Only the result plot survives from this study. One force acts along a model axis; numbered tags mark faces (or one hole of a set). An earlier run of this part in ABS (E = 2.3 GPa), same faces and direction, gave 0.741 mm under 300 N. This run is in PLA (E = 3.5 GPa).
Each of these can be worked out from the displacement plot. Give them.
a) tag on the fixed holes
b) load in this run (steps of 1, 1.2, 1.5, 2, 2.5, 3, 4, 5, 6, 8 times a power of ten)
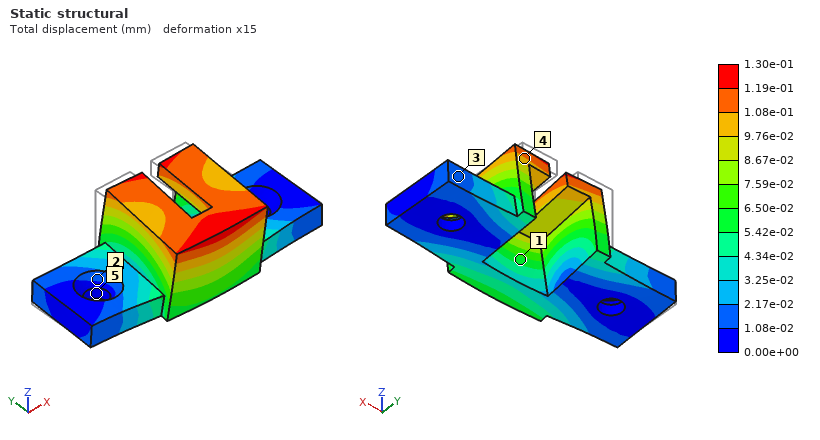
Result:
5
80 N
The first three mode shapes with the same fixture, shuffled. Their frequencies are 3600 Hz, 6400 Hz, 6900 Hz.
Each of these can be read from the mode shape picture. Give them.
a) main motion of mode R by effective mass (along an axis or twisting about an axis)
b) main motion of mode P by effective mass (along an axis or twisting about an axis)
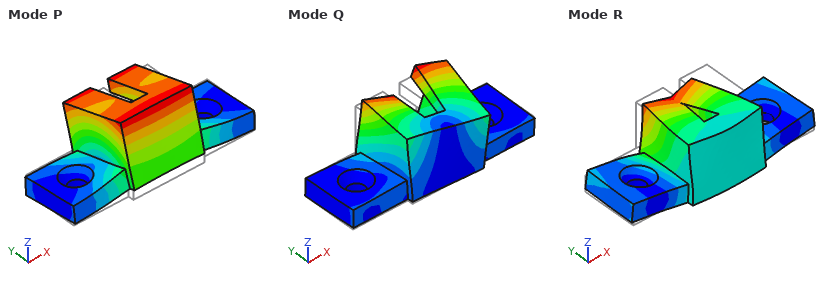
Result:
along Z
along Y
